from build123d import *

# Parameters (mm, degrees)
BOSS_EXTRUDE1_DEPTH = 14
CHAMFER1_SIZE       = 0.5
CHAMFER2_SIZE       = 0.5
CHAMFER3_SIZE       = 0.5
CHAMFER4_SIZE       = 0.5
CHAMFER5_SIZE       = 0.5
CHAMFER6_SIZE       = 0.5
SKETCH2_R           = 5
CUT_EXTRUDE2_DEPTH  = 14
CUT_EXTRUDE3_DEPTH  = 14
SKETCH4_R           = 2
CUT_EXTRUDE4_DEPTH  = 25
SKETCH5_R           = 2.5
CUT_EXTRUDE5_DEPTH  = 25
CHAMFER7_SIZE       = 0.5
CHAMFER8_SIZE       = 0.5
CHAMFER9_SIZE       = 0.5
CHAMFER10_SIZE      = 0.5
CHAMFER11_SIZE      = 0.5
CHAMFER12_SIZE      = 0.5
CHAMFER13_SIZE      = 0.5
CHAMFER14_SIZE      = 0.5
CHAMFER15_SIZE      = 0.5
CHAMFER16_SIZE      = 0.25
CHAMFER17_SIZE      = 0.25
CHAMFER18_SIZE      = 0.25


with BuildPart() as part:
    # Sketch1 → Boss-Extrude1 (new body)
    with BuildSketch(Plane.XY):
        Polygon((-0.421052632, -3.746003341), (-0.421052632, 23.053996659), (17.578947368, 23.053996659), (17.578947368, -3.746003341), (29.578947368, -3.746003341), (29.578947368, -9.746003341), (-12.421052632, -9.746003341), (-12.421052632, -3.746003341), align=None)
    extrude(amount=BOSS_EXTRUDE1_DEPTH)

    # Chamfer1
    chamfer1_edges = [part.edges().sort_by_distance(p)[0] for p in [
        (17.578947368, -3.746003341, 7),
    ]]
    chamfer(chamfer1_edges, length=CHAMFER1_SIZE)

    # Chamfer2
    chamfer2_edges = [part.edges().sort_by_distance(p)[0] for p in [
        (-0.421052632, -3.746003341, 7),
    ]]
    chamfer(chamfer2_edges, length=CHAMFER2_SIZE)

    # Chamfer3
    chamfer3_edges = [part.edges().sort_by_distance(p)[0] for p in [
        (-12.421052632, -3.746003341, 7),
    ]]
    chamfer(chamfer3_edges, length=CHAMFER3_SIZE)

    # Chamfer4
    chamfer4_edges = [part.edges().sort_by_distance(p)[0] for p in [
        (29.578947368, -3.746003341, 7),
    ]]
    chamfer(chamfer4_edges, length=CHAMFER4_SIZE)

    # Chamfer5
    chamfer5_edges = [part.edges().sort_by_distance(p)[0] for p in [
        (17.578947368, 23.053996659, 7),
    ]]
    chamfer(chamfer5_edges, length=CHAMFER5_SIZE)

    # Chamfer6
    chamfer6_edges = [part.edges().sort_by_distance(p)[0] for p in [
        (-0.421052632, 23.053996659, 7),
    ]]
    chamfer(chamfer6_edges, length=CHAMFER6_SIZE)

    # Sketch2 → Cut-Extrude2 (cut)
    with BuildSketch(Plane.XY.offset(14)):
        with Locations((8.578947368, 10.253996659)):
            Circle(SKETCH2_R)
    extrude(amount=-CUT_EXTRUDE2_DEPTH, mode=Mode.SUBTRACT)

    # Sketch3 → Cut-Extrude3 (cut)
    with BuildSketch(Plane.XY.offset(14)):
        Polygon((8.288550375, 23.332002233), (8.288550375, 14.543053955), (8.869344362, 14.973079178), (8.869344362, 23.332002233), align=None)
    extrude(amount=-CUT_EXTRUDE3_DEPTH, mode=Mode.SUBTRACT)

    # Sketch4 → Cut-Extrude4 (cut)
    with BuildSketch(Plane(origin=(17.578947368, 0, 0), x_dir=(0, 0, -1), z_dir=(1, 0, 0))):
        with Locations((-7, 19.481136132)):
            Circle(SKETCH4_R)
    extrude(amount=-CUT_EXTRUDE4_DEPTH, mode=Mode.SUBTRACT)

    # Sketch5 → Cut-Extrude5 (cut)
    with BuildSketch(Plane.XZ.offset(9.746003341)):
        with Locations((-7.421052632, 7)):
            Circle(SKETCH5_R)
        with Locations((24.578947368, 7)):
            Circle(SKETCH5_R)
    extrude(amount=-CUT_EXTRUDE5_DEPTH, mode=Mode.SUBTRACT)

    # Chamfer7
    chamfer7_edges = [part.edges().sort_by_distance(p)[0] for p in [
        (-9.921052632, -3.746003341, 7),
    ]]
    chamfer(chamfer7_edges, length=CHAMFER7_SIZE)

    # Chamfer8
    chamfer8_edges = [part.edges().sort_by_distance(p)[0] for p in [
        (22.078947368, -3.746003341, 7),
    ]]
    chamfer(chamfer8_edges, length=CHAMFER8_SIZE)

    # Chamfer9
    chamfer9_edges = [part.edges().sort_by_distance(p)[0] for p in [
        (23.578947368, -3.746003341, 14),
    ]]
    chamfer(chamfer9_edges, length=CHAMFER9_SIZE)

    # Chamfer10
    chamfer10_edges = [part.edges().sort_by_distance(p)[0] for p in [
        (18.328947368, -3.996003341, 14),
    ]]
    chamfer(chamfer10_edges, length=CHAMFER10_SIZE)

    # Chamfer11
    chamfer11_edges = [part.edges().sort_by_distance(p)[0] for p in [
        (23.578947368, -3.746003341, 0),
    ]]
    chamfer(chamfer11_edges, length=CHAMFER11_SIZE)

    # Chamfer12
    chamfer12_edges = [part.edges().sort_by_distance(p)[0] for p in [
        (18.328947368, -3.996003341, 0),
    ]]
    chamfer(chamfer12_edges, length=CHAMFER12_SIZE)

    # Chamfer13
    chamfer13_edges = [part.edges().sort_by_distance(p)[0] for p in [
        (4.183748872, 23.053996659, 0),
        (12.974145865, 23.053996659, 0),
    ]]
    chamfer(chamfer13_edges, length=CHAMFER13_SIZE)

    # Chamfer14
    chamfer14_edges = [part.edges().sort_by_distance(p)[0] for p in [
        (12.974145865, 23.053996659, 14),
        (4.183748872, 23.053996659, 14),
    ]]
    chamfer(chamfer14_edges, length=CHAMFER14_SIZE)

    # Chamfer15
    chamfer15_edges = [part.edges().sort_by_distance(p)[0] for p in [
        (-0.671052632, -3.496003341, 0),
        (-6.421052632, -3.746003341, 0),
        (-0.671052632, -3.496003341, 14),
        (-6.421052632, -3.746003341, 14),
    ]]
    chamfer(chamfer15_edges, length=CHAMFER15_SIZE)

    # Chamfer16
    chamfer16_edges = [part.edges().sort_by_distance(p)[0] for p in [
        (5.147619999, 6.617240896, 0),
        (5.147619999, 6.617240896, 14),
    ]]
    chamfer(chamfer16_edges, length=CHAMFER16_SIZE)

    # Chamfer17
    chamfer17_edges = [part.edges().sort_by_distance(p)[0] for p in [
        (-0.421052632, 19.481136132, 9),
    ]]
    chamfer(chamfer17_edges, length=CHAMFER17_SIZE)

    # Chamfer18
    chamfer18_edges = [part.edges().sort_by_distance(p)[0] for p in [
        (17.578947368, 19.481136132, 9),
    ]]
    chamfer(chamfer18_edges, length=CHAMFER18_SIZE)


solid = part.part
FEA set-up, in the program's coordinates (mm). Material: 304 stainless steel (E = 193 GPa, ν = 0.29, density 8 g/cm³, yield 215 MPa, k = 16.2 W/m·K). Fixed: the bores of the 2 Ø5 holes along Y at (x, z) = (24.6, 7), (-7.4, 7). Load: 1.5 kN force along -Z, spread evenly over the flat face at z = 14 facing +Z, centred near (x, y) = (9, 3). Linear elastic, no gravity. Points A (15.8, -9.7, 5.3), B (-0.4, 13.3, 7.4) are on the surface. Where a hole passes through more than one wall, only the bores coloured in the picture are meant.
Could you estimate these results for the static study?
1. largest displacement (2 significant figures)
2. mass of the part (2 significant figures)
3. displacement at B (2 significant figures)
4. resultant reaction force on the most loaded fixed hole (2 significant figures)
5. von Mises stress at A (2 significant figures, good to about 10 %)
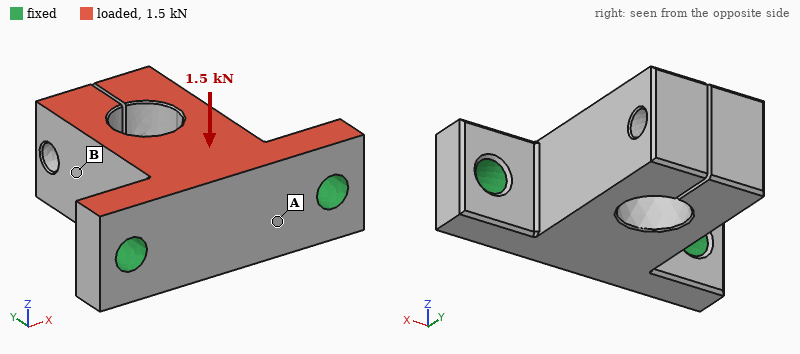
34 µm
69 g
21 µm
750 N
28 MPa
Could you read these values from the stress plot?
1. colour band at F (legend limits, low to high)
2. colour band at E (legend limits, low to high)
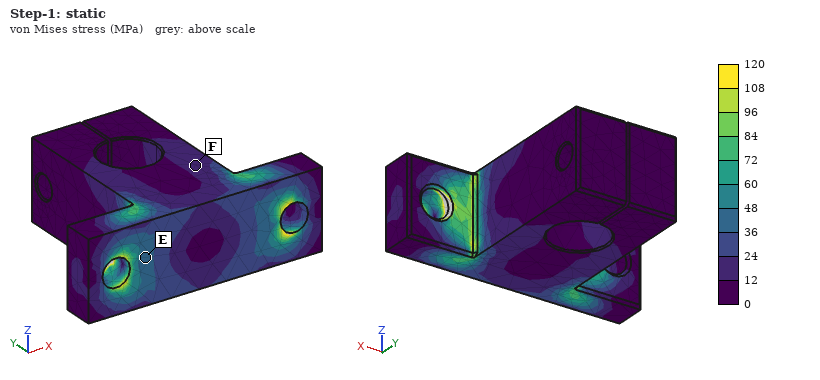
12 to 24 MPa
36 to 48 MPa
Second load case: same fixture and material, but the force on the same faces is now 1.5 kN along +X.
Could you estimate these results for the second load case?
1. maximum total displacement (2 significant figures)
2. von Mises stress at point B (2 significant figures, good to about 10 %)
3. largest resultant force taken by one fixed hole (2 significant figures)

23 µm
25 MPa
1.0 kN
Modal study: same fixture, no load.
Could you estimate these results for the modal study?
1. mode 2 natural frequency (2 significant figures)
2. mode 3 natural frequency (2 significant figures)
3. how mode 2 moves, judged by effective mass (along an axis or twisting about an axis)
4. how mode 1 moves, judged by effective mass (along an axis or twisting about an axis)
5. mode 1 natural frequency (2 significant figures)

6600 Hz
7300 Hz
along X
along Z
4900 Hz
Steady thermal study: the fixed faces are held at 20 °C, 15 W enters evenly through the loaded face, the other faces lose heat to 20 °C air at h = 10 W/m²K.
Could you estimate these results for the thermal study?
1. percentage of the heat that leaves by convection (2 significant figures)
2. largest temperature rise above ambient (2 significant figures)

10 %
79 K
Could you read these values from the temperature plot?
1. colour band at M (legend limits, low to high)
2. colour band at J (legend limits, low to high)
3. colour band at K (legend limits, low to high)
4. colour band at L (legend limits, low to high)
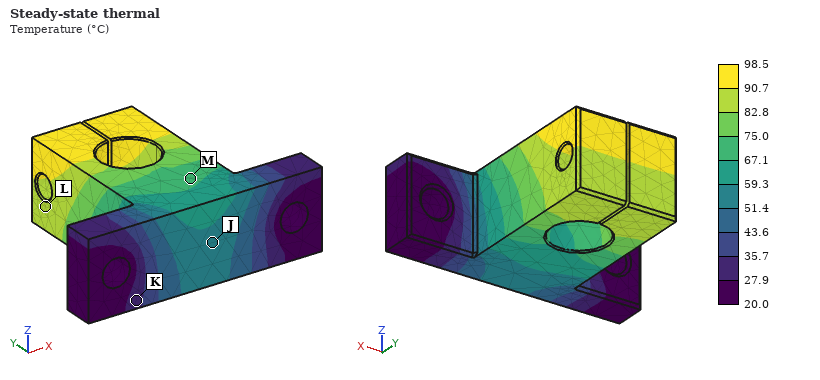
67.1 to 75.0 °C
51.4 to 59.3 °C
27.9 to 35.7 °C
82.8 to 90.7 °C
